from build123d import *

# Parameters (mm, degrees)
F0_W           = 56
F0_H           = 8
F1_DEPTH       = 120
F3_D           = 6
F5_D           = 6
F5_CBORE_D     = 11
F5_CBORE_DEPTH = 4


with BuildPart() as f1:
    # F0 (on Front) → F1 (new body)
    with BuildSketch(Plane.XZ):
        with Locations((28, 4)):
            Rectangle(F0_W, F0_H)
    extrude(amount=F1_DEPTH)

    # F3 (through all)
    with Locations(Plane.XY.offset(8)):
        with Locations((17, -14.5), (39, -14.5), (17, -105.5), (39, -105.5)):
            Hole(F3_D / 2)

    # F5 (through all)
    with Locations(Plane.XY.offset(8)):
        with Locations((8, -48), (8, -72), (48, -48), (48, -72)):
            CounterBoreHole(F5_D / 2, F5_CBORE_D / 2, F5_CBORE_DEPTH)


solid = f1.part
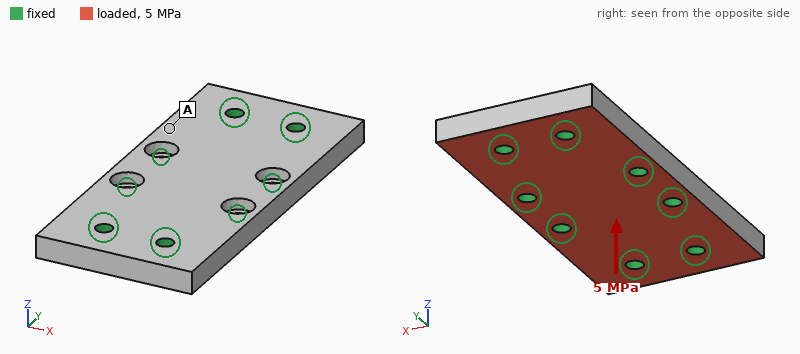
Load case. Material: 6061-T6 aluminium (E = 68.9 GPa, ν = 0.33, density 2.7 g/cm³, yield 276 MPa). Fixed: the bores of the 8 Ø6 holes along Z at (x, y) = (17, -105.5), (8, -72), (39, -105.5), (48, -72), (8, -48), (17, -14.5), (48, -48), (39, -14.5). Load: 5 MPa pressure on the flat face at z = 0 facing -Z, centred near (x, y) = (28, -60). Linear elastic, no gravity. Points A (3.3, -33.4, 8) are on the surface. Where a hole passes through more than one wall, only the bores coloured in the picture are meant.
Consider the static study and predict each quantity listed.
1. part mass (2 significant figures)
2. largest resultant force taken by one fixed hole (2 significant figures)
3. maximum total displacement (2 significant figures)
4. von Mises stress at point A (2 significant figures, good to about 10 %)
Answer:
140 g
4.5 kN
25 µm
27 MPa
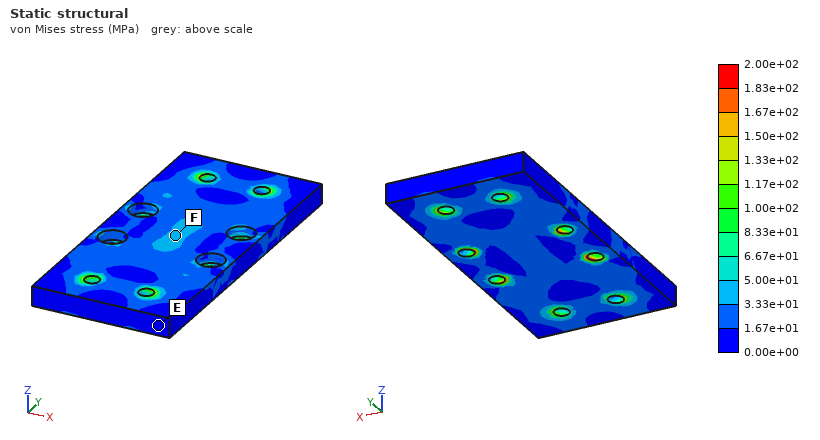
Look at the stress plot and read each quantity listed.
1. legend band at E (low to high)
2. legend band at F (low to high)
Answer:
0.00e+00 to 1.67e+01 MPa
3.33e+01 to 5.00e+01 MPa
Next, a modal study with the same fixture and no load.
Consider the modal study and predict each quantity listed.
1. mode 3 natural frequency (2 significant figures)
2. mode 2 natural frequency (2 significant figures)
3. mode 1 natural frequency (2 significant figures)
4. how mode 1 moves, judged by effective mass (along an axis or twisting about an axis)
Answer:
19 kHz
19 kHz
18 kHz
along Z
